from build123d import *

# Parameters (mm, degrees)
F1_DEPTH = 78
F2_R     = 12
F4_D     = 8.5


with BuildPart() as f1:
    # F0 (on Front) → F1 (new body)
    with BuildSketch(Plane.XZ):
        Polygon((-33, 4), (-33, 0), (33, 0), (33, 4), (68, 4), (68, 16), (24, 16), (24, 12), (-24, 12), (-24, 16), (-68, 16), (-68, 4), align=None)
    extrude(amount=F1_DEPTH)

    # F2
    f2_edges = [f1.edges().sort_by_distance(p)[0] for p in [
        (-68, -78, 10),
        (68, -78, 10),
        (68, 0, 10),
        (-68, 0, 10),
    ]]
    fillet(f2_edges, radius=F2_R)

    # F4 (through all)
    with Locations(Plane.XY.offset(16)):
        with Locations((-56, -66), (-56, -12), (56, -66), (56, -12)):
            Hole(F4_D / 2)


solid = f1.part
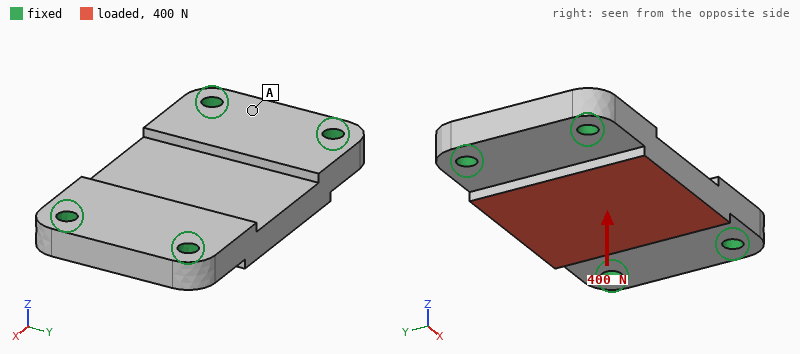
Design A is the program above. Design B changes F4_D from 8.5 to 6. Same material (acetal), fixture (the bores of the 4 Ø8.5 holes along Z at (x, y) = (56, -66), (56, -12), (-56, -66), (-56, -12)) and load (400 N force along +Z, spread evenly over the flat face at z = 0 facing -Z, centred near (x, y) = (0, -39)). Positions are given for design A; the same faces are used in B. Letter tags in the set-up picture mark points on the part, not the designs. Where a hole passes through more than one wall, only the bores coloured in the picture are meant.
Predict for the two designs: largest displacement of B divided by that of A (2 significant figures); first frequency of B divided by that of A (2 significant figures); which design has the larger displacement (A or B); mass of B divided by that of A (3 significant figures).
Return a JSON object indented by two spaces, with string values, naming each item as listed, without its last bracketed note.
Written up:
{
  "largest displacement of B divided by that of A": "1.1",
  "first frequency of B divided by that of A": "0.92",
  "which design has the larger displacement": "B",
  "mass of B divided by that of A": "1.01"
}
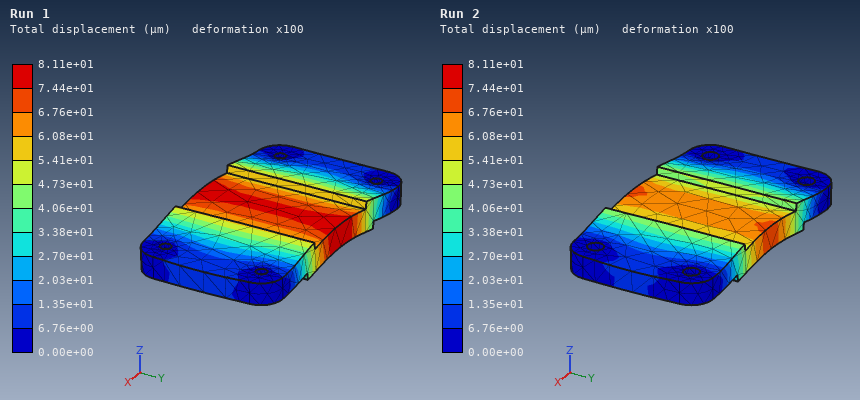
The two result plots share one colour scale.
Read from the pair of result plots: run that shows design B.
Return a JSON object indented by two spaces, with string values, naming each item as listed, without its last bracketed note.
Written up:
{
  "run that shows design B": "Run 1"
}
